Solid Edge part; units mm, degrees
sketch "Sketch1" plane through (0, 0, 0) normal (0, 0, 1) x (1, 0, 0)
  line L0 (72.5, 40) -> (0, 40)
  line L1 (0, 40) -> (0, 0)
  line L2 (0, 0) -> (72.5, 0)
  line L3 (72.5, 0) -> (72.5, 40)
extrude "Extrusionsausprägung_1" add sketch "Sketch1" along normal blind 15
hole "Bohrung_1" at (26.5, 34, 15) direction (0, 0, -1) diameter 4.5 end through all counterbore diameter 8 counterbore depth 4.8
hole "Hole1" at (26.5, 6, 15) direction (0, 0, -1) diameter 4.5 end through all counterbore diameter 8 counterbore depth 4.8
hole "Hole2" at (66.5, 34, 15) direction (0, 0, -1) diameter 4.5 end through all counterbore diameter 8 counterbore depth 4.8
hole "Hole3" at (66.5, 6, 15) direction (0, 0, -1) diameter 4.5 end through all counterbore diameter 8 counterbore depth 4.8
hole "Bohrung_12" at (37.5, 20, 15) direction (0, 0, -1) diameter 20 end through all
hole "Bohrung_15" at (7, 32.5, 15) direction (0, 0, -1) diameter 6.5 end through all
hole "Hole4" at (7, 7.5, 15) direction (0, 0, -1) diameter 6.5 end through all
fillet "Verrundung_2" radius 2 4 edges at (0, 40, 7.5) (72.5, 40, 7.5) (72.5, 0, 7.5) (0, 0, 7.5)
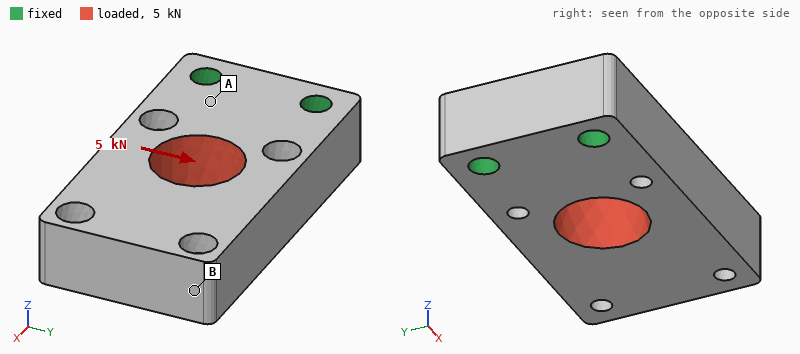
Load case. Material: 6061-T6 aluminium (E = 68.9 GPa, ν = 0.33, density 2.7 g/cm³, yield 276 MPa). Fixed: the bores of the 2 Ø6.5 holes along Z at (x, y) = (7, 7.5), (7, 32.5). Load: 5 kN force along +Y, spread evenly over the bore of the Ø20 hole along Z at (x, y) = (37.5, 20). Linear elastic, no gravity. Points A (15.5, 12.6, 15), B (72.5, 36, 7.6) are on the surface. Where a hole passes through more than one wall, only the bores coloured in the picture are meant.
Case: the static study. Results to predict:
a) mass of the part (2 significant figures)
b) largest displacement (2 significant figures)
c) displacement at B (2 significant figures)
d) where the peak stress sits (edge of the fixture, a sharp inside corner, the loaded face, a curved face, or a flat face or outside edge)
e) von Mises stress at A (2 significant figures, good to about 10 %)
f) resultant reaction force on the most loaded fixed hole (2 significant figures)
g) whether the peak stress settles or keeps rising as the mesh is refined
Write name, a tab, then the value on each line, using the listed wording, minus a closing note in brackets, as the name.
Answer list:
mass of the part	98 g
largest displacement	57 µm
displacement at B	57 µm
where the peak stress sits	edge of the fixture
von Mises stress at A	22 MPa
resultant reaction force on the most loaded fixed hole	5.7 kN
whether the peak stress settles or keeps rising as the mesh is refined	keeps rising
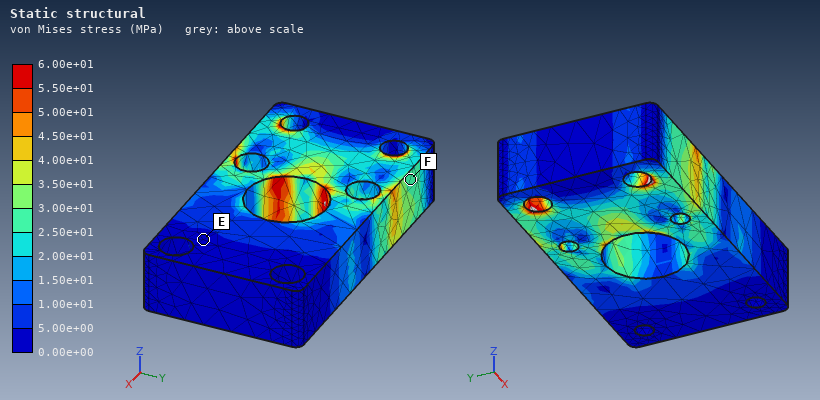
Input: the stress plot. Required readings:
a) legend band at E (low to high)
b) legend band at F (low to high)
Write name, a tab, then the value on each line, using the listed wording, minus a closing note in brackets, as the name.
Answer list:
legend band at E	0.00e+00 to 5.00e+00 MPa
legend band at F	2.50e+01 to 3.00e+01 MPa
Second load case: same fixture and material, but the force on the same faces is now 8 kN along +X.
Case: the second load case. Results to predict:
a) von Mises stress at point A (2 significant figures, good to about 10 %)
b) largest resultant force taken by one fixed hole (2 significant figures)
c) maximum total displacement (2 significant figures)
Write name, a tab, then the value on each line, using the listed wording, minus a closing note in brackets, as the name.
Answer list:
von Mises stress at point A	15 MPa
largest resultant force taken by one fixed hole	4.0 kN
maximum total displacement	16 µm
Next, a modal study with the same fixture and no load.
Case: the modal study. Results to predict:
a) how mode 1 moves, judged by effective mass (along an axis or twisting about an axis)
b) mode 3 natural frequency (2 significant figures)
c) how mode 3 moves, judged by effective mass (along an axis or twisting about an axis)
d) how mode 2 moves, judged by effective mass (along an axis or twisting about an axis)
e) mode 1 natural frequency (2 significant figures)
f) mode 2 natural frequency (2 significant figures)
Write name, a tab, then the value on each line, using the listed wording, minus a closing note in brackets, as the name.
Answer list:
how mode 1 moves, judged by effective mass	along Z
mode 3 natural frequency	7000 Hz
how mode 3 moves, judged by effective mass	twisting about X
how mode 2 moves, judged by effective mass	along Y
mode 1 natural frequency	2400 Hz
mode 2 natural frequency	5200 Hz
